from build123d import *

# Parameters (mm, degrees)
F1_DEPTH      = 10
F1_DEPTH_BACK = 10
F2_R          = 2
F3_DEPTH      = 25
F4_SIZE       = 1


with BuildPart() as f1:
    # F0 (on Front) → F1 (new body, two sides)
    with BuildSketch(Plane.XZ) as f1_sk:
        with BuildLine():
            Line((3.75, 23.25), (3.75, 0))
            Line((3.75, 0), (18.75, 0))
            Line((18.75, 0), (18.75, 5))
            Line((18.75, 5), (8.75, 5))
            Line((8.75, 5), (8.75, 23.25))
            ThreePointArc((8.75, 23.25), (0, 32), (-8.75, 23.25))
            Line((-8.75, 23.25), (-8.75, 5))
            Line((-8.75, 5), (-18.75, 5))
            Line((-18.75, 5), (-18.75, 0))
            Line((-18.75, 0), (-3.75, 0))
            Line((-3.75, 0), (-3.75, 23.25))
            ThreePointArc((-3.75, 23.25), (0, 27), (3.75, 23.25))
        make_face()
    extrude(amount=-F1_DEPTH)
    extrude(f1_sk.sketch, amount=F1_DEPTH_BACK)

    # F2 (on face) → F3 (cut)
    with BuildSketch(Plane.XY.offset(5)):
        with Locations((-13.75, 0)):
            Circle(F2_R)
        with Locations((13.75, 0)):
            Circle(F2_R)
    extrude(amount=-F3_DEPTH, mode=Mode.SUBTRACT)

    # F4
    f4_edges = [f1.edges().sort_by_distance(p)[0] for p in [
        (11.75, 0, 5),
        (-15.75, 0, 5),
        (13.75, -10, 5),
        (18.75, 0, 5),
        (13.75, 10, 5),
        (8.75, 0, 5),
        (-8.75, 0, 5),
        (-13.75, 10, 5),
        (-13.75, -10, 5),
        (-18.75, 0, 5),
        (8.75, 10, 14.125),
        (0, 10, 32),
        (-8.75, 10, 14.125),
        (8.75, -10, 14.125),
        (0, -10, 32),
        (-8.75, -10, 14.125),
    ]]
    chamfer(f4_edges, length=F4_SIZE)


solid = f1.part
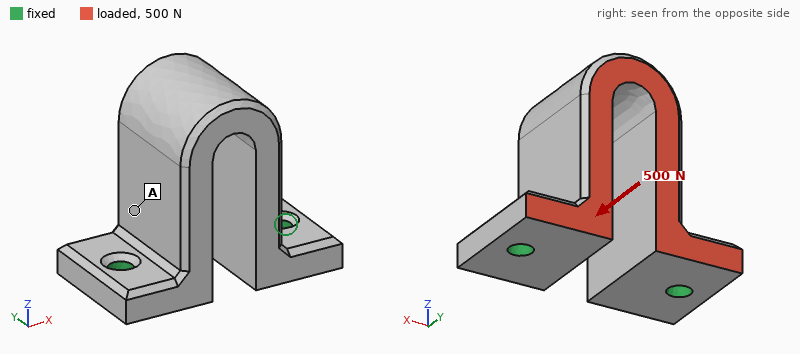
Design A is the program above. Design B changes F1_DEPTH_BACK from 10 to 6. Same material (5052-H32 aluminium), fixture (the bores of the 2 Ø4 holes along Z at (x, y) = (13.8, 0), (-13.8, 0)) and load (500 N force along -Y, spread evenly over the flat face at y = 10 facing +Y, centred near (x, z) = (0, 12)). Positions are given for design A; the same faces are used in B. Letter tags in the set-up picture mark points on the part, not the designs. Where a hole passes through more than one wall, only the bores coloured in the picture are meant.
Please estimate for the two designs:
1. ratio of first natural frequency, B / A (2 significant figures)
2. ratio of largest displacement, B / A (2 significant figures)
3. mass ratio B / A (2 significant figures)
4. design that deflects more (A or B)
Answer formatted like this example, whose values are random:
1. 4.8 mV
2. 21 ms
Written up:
1. 1.0
2. 1.2
3. 0.79
4. B
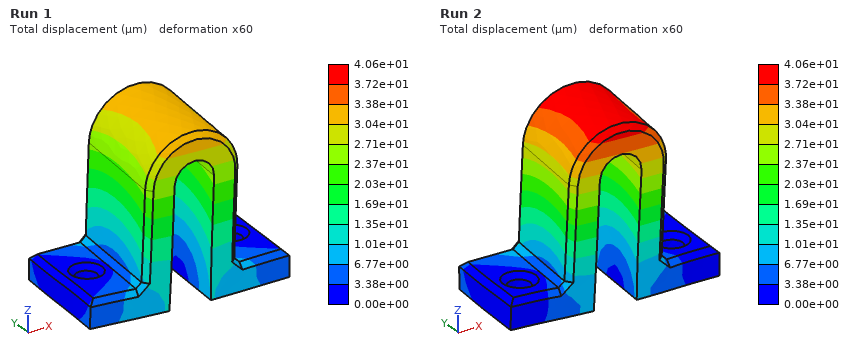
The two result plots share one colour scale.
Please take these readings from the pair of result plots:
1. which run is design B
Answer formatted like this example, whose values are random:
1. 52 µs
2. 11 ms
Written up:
1. Run 2
